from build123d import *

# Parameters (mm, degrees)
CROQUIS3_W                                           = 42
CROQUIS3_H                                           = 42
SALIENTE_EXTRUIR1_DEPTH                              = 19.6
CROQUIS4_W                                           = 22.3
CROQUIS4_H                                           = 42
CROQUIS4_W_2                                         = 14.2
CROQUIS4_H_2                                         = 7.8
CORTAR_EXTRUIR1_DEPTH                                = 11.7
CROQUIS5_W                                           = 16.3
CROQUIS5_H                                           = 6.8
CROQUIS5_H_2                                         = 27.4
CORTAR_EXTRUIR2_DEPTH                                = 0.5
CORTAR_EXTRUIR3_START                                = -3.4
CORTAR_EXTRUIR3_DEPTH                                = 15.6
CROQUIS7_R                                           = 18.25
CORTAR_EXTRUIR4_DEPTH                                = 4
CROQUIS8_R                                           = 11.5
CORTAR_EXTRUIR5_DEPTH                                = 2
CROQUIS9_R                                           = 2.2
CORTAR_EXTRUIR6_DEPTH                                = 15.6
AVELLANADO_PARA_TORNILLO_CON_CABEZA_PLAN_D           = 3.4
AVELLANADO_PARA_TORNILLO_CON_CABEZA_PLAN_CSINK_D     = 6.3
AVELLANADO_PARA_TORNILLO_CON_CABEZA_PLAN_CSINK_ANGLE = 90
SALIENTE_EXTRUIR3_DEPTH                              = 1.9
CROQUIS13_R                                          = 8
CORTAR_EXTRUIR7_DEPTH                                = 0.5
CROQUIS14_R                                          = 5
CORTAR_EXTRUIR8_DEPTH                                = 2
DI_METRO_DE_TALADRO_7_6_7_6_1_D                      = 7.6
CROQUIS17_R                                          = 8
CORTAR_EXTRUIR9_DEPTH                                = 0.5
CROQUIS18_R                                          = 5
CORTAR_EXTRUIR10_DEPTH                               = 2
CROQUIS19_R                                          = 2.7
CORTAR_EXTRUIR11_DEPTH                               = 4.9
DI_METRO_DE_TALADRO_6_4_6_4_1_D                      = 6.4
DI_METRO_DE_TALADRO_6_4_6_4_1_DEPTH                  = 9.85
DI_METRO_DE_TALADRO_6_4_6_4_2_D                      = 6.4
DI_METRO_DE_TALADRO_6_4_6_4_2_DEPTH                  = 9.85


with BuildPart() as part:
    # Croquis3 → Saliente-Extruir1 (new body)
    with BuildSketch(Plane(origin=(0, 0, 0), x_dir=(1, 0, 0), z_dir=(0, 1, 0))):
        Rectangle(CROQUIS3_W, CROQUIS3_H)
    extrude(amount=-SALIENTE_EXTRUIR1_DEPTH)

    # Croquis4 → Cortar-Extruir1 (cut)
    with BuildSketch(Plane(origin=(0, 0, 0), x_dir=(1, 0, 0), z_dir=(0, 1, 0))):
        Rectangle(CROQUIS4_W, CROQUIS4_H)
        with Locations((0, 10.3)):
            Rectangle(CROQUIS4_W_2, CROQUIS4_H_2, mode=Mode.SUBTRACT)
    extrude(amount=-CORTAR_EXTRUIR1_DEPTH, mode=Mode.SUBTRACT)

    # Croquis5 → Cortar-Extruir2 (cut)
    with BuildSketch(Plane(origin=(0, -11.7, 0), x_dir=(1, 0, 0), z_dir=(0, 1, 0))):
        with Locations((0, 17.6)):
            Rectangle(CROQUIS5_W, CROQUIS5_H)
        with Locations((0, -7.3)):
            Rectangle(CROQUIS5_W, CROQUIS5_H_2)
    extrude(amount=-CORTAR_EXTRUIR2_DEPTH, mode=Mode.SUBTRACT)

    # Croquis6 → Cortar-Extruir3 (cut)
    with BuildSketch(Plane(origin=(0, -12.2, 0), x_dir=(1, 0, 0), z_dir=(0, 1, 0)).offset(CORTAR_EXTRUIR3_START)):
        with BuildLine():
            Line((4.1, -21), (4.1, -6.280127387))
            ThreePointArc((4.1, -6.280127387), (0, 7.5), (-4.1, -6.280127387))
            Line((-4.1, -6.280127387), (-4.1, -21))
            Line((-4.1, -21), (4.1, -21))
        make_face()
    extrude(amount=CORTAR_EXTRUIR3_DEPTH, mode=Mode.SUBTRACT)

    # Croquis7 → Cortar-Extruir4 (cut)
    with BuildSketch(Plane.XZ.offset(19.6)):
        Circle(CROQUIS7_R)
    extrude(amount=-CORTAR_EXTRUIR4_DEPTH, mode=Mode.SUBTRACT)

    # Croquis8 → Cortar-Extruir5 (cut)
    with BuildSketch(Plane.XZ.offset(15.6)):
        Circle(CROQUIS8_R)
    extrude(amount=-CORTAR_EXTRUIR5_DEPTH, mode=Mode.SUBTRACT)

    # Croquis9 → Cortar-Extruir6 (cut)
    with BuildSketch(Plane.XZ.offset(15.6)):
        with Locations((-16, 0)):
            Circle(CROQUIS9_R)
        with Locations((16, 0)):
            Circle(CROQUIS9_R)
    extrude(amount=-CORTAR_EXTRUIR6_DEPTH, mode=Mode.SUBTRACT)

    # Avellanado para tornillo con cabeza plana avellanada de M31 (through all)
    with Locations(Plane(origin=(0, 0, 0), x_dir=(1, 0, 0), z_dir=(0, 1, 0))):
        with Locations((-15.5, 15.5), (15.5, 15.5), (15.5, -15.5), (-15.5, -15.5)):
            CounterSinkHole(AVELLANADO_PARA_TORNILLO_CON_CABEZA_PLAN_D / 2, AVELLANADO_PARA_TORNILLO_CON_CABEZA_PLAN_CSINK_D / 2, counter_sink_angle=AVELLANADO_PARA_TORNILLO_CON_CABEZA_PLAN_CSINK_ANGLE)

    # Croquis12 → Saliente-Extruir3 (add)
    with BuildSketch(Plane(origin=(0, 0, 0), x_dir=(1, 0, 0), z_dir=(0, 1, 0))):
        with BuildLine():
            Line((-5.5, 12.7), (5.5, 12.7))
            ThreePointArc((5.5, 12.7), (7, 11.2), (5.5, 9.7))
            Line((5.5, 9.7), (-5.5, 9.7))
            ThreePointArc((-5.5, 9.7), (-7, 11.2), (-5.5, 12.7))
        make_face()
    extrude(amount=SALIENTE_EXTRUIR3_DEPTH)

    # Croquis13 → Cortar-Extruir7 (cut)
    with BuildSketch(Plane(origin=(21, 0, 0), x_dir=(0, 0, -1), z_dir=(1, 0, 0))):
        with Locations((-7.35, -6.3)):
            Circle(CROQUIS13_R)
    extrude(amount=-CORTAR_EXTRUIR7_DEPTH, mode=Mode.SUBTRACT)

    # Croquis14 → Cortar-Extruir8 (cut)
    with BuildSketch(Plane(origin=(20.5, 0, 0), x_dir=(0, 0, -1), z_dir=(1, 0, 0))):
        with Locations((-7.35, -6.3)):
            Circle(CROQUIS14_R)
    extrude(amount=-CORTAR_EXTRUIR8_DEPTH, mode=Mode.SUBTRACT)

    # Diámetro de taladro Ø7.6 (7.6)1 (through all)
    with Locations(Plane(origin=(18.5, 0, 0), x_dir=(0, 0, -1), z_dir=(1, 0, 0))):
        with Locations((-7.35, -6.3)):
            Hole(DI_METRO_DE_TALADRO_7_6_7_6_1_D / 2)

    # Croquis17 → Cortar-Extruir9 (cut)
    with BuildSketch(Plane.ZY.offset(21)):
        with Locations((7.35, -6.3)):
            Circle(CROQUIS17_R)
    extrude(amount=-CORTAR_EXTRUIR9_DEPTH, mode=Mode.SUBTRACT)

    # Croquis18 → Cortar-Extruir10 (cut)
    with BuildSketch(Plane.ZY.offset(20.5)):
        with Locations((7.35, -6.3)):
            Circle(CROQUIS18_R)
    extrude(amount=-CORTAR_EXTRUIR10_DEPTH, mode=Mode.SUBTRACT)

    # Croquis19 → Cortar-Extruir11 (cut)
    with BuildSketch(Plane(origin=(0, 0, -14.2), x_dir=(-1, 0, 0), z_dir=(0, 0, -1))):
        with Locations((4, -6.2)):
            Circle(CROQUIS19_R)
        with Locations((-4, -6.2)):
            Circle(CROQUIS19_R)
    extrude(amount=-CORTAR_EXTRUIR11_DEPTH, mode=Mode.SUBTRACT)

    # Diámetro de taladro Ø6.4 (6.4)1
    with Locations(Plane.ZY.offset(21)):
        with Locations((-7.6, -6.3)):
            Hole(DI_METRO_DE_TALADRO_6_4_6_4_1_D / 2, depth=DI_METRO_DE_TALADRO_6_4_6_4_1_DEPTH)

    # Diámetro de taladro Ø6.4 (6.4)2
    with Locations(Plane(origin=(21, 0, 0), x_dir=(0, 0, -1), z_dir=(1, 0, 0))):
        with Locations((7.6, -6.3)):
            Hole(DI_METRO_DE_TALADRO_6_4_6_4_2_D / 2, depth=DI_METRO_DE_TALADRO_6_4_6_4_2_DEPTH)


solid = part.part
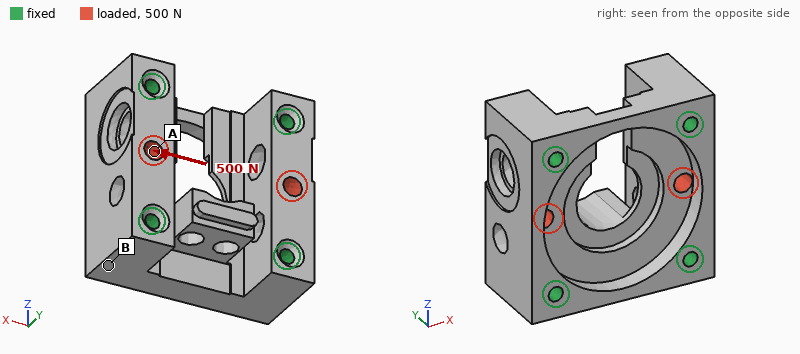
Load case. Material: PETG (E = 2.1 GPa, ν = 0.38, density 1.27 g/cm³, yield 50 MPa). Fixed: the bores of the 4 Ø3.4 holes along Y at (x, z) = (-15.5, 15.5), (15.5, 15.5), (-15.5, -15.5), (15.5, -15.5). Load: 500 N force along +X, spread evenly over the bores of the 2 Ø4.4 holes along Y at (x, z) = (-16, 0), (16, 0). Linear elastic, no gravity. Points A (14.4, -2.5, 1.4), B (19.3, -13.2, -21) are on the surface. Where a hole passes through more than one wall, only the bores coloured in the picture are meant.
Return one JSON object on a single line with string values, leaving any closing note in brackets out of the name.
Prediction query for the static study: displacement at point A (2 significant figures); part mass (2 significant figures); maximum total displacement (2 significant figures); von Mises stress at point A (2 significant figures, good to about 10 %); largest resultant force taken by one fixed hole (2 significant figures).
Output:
{"displacement at point A": "52 µm", "part mass": "20 g", "maximum total displacement": "56 µm", "von Mises stress at point A": "1.4 MPa", "largest resultant force taken by one fixed hole": "140 N"}
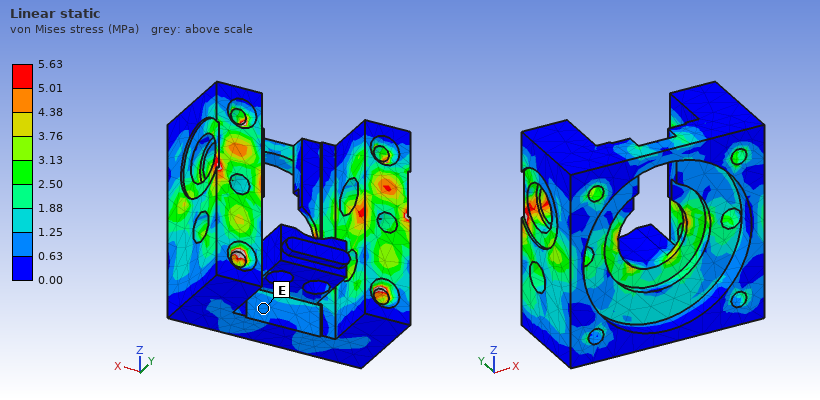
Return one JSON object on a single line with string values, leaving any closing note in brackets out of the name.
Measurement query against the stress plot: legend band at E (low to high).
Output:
{"legend band at E": "0.63 to 1.25 MPa"}
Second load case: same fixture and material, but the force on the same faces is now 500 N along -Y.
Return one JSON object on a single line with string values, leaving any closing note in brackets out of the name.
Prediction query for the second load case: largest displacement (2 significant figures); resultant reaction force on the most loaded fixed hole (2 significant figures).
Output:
{"largest displacement": "40 µm", "resultant reaction force on the most loaded fixed hole": "140 N"}
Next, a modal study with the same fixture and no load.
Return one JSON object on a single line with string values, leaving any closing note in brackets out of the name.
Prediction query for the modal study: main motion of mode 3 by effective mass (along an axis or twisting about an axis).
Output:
{"main motion of mode 3 by effective mass": "along Y"}
